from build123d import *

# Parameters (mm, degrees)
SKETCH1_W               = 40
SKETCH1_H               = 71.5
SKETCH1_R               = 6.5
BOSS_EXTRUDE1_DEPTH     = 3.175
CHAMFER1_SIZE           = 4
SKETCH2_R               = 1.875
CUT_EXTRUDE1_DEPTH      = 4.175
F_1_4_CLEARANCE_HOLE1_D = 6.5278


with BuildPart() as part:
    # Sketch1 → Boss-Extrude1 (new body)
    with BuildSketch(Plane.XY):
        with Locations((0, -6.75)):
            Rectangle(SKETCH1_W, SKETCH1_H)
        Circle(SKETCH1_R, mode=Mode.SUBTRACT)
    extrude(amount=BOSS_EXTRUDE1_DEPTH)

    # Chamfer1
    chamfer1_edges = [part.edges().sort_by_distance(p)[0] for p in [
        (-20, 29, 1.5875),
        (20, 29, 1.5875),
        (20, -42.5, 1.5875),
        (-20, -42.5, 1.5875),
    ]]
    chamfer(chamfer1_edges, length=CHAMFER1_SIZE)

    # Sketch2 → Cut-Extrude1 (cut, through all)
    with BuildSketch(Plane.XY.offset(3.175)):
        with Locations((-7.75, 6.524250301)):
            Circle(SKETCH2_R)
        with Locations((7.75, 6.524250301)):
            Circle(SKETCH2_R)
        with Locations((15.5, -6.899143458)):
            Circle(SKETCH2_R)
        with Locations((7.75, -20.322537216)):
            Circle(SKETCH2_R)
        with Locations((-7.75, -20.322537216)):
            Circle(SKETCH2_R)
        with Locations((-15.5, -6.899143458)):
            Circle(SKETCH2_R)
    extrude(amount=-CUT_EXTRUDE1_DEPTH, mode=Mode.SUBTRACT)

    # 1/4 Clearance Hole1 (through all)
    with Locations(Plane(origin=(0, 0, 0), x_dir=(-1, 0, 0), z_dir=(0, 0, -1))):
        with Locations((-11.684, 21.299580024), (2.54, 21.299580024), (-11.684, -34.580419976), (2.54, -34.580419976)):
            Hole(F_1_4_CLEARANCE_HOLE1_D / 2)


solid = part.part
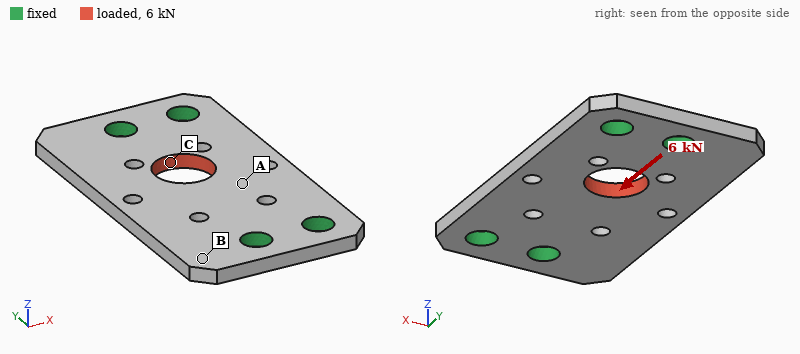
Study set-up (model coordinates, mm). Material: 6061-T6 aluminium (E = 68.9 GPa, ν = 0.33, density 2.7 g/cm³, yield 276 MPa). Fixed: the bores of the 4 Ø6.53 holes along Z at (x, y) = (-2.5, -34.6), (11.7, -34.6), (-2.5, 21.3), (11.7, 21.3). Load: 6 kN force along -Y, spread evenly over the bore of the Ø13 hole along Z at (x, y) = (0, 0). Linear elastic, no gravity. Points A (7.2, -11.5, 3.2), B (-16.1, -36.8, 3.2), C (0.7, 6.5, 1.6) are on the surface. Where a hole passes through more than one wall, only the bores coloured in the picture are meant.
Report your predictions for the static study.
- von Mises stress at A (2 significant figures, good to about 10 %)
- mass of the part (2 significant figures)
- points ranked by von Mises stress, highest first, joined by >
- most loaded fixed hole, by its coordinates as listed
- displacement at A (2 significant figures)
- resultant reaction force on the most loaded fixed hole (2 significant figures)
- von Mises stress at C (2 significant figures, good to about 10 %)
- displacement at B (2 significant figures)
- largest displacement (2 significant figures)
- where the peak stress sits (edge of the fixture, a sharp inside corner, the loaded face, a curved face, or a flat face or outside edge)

31 MPa
21 g
C > A > B
(-2.5, 21.3)
9.4 µm
2.1 kN
54 MPa
6.3 µm
18 µm
a curved face
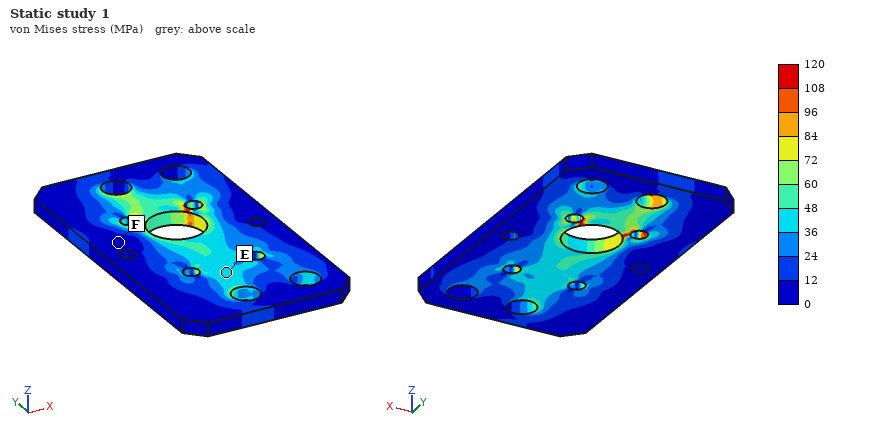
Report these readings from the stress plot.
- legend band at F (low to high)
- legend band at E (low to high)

0 to 12 MPa
36 to 48 MPa
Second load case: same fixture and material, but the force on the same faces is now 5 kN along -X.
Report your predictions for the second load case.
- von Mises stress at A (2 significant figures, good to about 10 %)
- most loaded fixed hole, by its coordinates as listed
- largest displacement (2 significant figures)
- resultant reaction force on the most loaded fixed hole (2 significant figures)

38 MPa
(-2.5, 21.3)
32 µm
1.9 kN
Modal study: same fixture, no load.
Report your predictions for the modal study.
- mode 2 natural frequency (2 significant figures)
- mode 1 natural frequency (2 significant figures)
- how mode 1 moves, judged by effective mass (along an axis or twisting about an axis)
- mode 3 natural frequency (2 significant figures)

6800 Hz
5200 Hz
along Z
10 kHz
